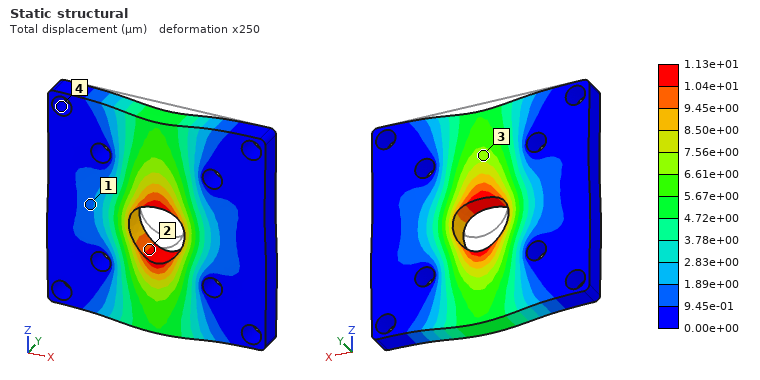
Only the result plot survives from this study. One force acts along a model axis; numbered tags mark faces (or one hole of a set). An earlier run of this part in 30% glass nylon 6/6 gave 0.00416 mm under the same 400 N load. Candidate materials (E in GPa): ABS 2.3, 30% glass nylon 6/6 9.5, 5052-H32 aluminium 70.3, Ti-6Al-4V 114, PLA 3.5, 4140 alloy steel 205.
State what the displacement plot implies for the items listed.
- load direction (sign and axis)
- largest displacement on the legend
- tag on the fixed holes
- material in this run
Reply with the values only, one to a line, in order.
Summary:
-Z
1.13e+01 µm
4
PLA
